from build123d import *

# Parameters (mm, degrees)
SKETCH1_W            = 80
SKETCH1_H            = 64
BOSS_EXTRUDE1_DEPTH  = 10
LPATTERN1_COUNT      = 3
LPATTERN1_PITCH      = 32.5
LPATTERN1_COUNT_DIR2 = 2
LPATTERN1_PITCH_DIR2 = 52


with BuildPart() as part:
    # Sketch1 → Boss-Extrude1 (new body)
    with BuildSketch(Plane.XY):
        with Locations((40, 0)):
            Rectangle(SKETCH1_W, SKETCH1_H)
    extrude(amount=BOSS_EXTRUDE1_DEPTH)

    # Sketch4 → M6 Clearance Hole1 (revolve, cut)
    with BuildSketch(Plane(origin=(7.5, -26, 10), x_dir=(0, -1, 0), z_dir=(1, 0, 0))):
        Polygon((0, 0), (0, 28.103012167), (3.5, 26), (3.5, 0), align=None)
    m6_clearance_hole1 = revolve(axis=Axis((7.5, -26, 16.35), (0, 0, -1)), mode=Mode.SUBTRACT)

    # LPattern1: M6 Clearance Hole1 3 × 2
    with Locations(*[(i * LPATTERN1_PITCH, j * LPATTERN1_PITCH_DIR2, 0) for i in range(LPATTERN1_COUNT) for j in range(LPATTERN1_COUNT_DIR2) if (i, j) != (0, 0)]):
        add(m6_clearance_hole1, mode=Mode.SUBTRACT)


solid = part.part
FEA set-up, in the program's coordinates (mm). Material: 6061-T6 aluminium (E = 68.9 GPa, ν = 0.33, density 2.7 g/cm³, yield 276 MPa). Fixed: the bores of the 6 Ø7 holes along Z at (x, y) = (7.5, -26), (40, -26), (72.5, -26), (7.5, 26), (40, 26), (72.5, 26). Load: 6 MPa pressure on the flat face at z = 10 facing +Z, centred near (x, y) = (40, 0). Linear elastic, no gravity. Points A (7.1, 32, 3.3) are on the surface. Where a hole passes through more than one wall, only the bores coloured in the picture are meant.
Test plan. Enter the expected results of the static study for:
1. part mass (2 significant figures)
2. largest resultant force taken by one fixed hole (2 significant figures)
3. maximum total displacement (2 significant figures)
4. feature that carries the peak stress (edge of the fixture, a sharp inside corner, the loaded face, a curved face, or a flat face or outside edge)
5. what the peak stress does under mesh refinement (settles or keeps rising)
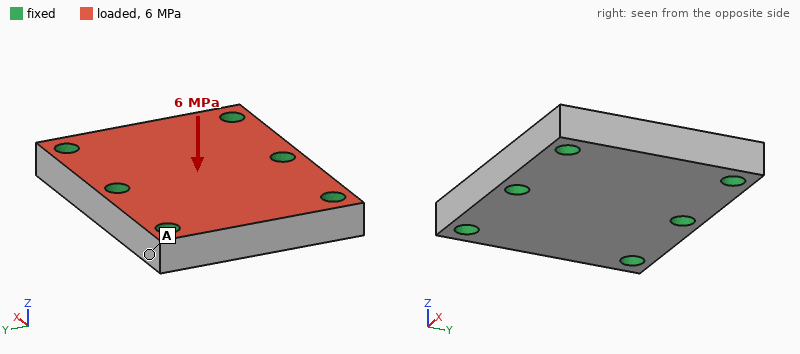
130 g
6.1 kN
31 µm
edge of the fixture
keeps rising
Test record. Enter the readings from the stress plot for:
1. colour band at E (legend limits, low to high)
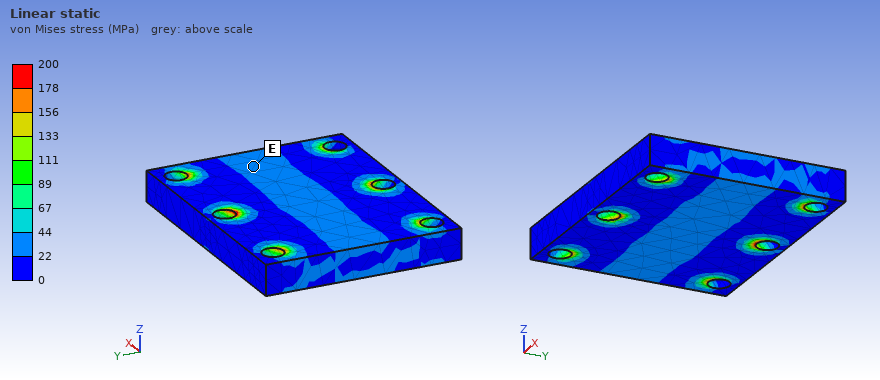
22 to 44 MPa
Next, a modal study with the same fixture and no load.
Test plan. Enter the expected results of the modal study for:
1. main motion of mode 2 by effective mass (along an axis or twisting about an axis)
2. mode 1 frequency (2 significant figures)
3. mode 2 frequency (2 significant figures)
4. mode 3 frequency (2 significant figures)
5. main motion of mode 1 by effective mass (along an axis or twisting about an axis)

twisting about Y
15 kHz
18 kHz
22 kHz
along Z
